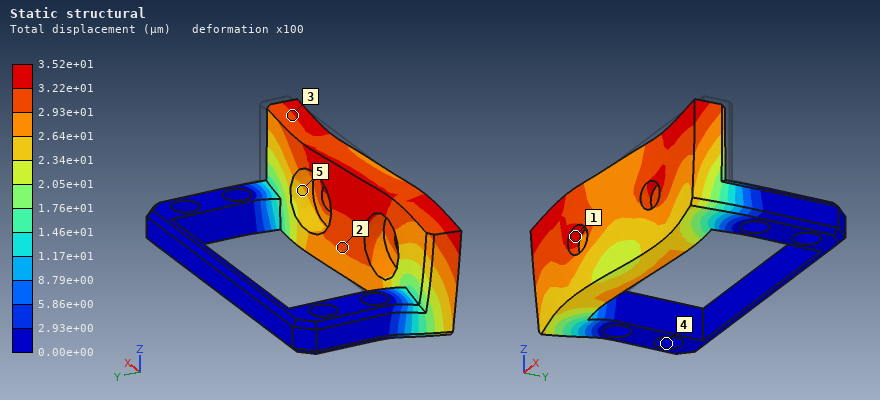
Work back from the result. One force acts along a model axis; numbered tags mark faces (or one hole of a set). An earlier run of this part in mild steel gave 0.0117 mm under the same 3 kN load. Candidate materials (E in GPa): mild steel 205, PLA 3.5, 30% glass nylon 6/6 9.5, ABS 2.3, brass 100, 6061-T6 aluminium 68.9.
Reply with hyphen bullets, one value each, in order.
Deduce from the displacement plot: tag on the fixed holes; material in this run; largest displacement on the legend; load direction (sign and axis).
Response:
- 4
- 6061-T6 aluminium
- 3.52e+01 µm
- -X
